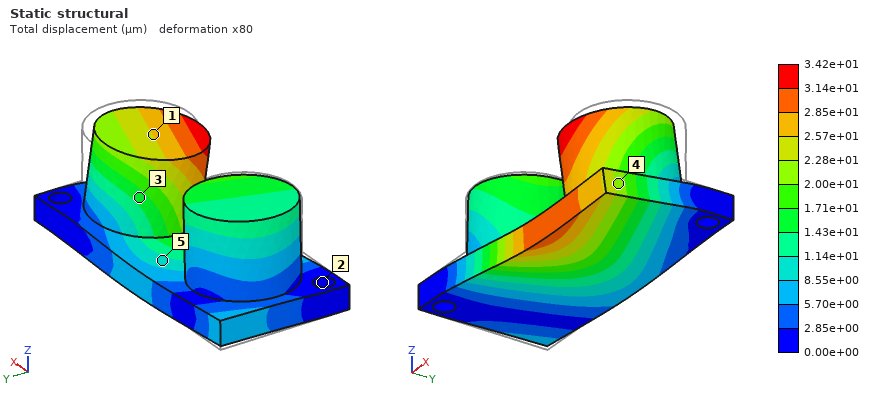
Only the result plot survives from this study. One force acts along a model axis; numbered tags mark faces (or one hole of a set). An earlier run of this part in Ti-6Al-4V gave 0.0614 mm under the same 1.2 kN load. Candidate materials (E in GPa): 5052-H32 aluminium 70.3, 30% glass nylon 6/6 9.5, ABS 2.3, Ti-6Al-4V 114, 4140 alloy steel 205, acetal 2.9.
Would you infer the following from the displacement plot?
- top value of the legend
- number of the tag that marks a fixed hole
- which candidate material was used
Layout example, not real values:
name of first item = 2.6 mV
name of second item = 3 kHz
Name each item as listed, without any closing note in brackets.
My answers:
top value of the legend = 3.42e+01 µm
number of the tag that marks a fixed hole = 2
which candidate material was used = 4140 alloy steel
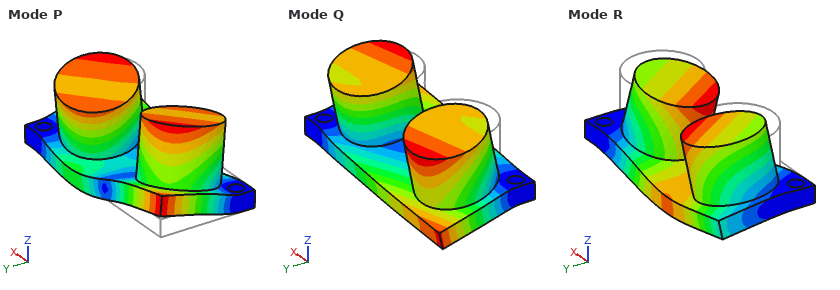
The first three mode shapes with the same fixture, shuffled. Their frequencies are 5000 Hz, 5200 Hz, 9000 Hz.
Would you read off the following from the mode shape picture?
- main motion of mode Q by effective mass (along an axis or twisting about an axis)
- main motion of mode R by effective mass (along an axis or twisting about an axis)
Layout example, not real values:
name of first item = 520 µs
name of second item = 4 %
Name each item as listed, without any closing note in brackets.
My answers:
main motion of mode Q by effective mass = along Y
main motion of mode R by effective mass = along Z
